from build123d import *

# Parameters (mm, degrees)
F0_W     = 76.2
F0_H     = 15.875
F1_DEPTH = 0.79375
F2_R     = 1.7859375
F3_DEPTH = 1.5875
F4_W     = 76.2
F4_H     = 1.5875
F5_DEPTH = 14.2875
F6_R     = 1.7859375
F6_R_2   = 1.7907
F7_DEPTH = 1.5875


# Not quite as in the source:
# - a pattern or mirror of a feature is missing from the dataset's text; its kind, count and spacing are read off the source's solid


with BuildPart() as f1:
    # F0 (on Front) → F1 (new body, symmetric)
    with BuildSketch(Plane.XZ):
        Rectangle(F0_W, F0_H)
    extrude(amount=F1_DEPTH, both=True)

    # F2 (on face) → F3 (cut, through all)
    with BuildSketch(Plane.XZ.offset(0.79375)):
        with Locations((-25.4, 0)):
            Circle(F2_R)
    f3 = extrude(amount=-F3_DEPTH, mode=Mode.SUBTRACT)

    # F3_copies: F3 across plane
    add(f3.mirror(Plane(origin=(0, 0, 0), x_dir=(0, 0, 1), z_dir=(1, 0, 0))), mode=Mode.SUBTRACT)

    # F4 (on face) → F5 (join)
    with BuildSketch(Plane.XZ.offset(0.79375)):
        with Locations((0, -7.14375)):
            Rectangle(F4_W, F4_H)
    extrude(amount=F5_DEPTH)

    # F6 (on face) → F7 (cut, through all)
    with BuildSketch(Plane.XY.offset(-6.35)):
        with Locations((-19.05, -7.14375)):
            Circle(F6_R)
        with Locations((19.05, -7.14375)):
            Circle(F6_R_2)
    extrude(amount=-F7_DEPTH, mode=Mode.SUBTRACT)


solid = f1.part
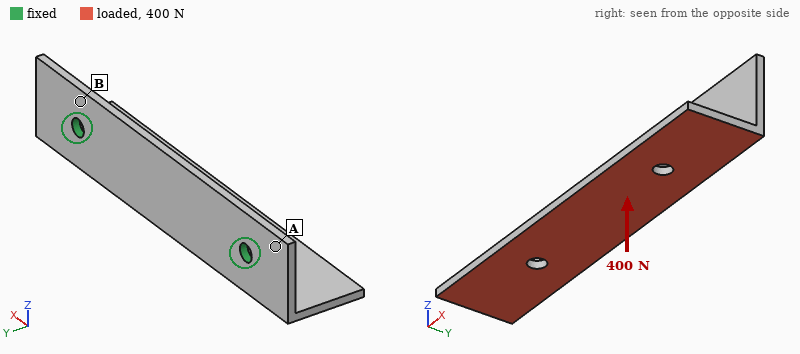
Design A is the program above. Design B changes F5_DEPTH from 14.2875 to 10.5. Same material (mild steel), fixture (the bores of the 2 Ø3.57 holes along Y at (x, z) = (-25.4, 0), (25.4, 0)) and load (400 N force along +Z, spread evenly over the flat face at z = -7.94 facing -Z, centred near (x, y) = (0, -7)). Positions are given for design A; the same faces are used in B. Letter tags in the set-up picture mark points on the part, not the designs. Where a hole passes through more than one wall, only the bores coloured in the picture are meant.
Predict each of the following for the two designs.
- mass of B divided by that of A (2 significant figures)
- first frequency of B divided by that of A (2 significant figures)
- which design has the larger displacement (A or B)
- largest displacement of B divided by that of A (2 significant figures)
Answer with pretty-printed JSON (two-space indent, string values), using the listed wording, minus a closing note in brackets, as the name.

{
  "mass of B divided by that of A": "0.87",
  "first frequency of B divided by that of A": "1.4",
  "which design has the larger displacement": "A",
  "largest displacement of B divided by that of A": "0.55"
}
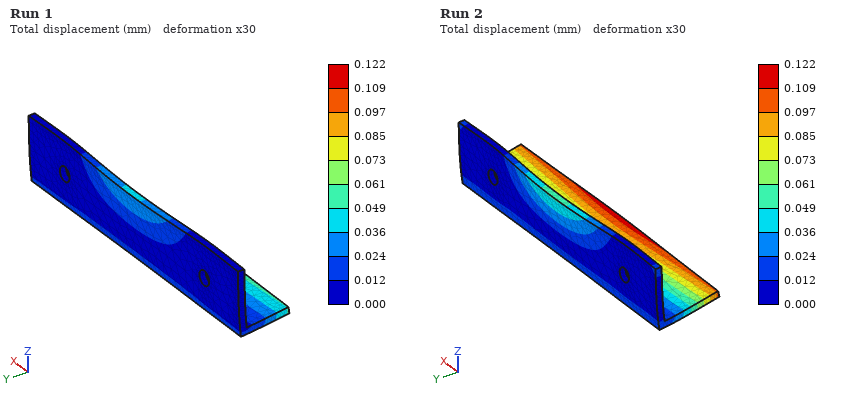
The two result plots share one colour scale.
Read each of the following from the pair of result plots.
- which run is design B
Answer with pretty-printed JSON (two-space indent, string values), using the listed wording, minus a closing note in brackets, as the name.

{
  "which run is design B": "Run 1"
}
